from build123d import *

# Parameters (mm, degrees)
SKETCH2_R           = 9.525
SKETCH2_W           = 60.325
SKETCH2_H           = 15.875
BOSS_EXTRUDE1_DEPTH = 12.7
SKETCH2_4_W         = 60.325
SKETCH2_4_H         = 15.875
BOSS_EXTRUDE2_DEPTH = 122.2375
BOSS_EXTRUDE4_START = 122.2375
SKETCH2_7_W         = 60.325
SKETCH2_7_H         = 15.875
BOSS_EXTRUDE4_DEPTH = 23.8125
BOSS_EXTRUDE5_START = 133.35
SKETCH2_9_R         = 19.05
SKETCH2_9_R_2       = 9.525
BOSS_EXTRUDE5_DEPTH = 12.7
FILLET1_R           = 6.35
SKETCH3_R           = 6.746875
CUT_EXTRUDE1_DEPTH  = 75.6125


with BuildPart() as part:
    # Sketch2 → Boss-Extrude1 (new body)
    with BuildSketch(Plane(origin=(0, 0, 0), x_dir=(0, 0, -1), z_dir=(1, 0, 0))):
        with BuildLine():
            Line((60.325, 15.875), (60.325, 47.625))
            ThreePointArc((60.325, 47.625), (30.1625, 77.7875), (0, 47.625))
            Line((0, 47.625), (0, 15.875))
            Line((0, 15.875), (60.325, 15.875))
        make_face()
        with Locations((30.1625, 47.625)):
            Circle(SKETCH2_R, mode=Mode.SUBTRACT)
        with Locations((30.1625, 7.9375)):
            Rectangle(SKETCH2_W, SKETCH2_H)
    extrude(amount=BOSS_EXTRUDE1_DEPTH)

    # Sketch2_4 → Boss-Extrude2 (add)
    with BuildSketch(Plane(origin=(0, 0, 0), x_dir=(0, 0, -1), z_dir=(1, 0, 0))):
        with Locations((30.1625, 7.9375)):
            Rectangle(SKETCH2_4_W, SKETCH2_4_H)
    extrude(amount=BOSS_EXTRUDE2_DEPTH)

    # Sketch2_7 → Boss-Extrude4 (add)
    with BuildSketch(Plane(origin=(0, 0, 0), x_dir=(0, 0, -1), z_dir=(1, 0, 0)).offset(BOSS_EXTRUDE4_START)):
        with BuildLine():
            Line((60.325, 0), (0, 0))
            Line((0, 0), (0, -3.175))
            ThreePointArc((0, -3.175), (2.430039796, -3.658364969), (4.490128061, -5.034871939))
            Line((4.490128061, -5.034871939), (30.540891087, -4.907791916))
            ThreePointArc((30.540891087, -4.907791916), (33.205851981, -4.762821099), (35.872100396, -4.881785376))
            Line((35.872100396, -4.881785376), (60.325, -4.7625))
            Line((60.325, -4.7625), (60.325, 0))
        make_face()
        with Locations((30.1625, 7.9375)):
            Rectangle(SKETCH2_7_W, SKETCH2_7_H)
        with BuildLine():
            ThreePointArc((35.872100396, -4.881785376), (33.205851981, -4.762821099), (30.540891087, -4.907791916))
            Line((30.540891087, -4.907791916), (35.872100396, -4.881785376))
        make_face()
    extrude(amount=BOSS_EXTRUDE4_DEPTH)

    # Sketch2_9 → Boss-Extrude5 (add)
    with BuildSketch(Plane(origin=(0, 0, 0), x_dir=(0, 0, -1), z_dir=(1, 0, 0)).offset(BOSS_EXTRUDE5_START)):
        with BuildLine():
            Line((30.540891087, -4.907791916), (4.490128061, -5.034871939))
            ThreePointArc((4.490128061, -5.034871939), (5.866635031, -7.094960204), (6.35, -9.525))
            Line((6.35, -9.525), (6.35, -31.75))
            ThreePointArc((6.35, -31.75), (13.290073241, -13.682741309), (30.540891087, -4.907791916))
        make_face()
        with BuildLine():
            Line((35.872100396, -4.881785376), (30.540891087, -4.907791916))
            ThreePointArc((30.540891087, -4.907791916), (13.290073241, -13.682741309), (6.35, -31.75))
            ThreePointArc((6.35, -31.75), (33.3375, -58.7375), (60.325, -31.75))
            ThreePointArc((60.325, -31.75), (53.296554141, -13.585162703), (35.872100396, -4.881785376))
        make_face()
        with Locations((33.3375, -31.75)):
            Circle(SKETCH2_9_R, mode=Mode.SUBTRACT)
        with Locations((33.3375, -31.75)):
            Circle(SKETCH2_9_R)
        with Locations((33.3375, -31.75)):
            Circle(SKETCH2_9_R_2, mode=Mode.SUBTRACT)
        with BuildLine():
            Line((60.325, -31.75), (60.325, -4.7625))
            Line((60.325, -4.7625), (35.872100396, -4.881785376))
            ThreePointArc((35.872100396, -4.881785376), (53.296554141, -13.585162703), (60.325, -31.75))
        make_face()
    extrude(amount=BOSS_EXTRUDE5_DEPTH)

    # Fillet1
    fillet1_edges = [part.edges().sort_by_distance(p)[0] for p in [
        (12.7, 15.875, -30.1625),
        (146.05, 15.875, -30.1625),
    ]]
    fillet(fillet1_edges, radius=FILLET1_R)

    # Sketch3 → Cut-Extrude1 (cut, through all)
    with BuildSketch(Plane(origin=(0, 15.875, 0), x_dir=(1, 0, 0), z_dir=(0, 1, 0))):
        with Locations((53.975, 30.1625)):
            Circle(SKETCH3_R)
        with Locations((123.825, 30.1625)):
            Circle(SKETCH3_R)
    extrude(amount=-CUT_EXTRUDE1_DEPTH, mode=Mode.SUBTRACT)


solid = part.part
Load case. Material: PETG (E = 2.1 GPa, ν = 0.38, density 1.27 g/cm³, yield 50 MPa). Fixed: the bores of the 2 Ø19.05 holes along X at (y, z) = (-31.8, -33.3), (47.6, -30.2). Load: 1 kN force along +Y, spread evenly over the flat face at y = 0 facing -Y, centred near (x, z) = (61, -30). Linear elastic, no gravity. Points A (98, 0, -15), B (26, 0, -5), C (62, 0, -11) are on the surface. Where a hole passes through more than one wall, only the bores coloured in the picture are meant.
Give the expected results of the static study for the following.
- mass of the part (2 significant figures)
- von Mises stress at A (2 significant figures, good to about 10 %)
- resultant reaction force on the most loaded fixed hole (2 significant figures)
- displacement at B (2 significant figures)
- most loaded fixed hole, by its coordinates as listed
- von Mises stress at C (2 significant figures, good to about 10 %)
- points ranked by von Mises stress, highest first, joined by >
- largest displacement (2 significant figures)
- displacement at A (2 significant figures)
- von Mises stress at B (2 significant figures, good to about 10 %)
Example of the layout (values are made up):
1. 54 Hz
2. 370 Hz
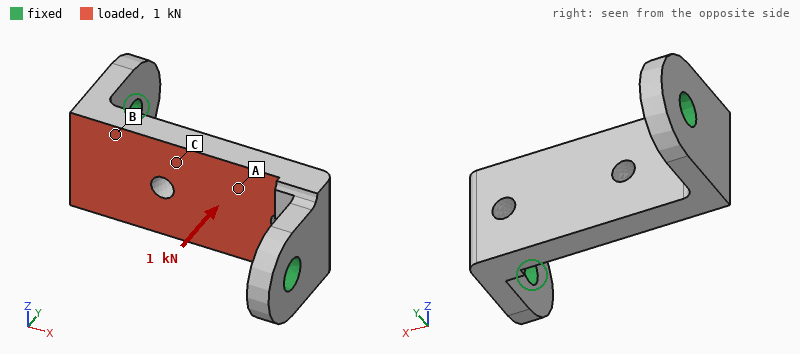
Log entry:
1. 270 g
2. 3.1 MPa
3. 600 N
4. 0.33 mm
5. (47.6, -30.2)
6. 4.5 MPa
7. C > A > B
8. 0.52 mm
9. 0.39 mm
10. 0.96 MPa
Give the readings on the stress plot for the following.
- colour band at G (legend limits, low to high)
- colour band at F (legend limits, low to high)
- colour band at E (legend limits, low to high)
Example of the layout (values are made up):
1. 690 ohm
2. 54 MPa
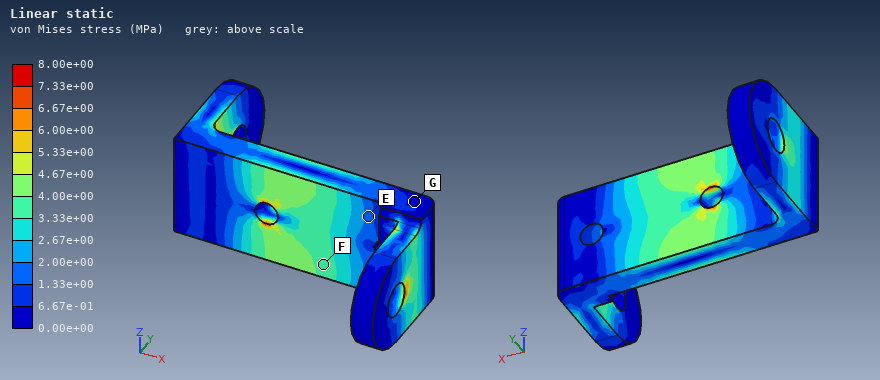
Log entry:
1. 0.00e+00 to 6.67e-01 MPa
2. 3.33e+00 to 4.00e+00 MPa
3. 1.33e+00 to 2.00e+00 MPa
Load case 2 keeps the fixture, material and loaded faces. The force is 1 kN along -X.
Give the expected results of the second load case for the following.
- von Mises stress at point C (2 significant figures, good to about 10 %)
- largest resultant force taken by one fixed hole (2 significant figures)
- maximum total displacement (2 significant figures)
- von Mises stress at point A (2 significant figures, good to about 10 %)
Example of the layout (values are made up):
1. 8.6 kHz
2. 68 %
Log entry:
1. 2.3 MPa
2. 510 N
3. 0.39 mm
4. 2.4 MPa
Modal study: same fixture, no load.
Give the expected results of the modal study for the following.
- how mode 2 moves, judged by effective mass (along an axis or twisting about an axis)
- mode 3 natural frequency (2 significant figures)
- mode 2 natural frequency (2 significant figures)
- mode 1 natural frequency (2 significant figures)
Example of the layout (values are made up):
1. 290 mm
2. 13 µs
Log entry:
1. along Z
2. 1200 Hz
3. 1000 Hz
4. 560 Hz
